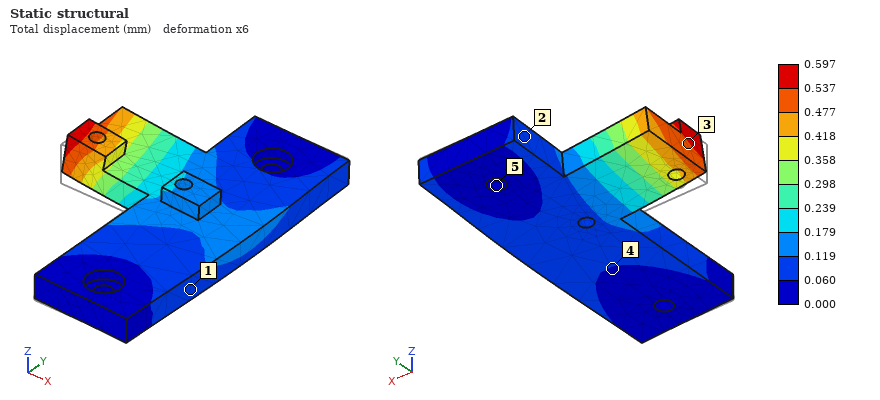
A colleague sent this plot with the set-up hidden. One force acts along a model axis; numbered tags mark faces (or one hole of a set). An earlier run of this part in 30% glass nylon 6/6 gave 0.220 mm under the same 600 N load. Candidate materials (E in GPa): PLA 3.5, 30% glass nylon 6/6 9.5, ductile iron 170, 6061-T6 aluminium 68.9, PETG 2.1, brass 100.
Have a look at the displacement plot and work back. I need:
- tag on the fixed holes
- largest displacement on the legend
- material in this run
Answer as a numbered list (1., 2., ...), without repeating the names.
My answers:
1. 5
2. 0.597 mm
3. PLA
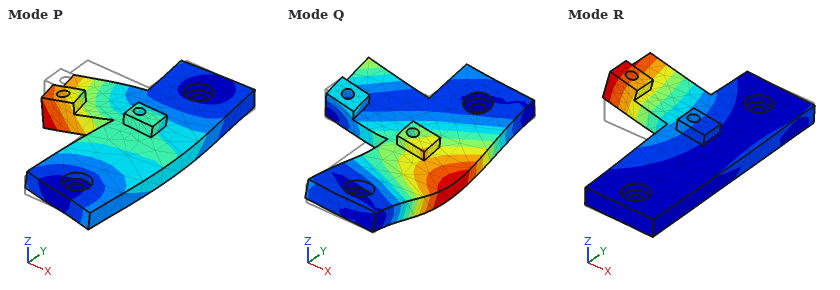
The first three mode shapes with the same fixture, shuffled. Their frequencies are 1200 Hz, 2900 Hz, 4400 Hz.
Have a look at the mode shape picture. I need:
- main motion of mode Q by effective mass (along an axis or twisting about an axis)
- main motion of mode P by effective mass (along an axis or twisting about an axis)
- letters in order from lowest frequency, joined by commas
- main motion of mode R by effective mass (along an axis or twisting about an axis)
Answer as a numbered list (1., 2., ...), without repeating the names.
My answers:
1. along Z
2. along X
3. R, Q, P
4. along Z
